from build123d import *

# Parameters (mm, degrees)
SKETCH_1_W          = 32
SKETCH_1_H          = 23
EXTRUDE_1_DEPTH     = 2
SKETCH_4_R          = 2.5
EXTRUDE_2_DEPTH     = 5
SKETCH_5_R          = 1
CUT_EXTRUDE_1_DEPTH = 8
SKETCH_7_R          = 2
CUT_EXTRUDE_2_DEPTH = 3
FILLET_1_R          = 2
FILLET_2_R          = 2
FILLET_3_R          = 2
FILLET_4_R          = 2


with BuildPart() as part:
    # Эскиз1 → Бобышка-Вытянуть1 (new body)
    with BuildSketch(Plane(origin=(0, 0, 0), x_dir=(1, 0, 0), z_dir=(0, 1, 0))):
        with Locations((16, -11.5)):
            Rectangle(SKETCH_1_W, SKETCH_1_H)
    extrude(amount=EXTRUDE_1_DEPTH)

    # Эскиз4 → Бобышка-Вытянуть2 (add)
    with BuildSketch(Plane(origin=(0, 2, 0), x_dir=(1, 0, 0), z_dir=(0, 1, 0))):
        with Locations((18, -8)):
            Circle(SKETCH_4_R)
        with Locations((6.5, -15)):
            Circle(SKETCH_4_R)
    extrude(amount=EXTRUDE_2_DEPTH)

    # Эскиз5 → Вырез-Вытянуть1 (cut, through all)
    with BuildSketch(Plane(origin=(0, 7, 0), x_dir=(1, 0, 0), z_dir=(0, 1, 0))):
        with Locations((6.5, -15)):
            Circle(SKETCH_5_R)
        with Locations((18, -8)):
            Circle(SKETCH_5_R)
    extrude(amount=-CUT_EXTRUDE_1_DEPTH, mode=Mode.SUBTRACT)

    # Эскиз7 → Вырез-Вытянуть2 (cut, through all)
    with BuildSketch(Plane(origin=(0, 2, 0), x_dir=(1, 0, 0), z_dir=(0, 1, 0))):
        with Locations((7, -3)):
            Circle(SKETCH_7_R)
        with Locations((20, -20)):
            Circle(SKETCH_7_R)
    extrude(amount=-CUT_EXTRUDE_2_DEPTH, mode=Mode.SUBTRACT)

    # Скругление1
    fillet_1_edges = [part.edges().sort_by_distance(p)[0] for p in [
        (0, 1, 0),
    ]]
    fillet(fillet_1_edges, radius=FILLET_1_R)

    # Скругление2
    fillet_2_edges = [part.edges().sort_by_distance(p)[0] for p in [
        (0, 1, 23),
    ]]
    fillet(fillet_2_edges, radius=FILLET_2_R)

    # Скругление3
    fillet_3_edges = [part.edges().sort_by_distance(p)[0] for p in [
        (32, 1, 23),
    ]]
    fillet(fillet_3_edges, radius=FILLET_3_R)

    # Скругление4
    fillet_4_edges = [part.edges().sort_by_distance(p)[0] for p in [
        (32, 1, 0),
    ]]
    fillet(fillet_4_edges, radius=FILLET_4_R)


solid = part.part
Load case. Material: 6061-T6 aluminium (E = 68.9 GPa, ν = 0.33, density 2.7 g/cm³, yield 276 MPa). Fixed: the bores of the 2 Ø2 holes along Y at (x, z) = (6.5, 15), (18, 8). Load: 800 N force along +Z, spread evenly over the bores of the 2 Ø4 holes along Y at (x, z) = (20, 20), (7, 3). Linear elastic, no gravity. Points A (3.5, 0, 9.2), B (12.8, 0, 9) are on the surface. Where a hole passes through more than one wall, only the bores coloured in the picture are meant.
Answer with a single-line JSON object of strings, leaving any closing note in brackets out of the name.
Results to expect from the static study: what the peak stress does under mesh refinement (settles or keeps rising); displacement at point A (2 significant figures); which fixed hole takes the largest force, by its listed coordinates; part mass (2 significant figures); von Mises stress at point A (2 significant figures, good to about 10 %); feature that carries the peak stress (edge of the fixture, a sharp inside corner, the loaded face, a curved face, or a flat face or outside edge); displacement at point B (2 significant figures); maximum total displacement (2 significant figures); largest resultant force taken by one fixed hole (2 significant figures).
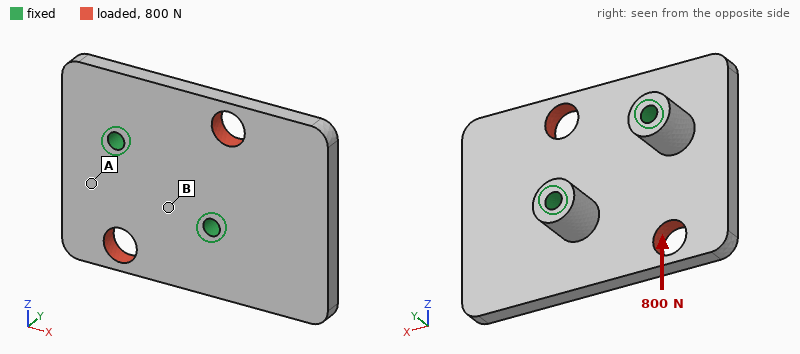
{"what the peak stress does under mesh refinement": "keeps rising", "displacement at point A": "2.1 µm", "which fixed hole takes the largest force, by its listed coordinates": "(18, 8)", "part mass": "4.2 g", "von Mises stress at point A": "16 MPa", "feature that carries the peak stress": "edge of the fixture", "displacement at point B": "1.6 µm", "maximum total displacement": "8.1 µm", "largest resultant force taken by one fixed hole": "460 N"}
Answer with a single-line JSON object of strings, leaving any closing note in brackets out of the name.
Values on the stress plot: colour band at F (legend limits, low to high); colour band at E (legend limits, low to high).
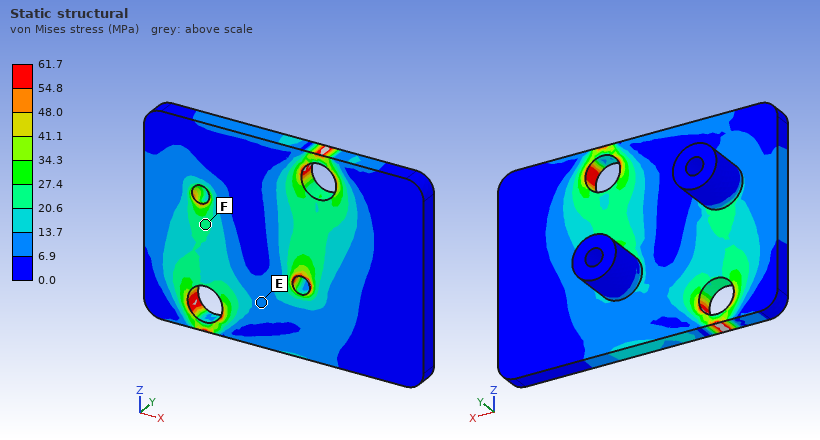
{"colour band at F": "20.6 to 27.4 MPa", "colour band at E": "6.9 to 13.7 MPa"}
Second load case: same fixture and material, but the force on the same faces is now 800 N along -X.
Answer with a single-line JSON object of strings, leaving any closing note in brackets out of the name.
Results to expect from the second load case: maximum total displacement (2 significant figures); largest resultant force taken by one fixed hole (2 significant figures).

{"maximum total displacement": "8.0 µm", "largest resultant force taken by one fixed hole": "420 N"}
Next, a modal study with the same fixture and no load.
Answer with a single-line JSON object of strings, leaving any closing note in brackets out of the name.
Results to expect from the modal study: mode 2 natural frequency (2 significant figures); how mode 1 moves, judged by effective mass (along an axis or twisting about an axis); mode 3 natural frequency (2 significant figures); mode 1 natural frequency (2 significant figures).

{"mode 2 natural frequency": "10 kHz", "how mode 1 moves, judged by effective mass": "along Y", "mode 3 natural frequency": "12 kHz", "mode 1 natural frequency": "6600 Hz"}
